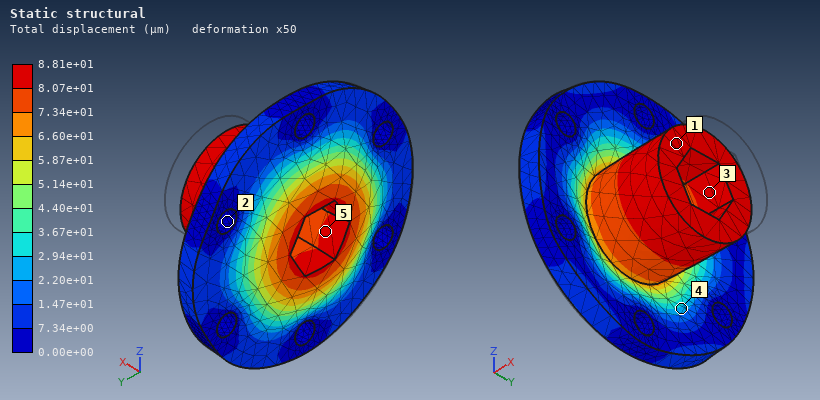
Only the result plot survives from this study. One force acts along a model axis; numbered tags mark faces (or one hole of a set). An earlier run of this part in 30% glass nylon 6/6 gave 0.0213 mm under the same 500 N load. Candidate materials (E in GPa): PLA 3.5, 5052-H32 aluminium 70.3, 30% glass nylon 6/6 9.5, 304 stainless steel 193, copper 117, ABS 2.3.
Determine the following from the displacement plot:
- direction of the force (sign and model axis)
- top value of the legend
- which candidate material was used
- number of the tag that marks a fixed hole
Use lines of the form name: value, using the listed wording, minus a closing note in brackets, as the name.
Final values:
direction of the force: -X
top value of the legend: 8.81e+01 µm
which candidate material was used: ABS
number of the tag that marks a fixed hole: 2
